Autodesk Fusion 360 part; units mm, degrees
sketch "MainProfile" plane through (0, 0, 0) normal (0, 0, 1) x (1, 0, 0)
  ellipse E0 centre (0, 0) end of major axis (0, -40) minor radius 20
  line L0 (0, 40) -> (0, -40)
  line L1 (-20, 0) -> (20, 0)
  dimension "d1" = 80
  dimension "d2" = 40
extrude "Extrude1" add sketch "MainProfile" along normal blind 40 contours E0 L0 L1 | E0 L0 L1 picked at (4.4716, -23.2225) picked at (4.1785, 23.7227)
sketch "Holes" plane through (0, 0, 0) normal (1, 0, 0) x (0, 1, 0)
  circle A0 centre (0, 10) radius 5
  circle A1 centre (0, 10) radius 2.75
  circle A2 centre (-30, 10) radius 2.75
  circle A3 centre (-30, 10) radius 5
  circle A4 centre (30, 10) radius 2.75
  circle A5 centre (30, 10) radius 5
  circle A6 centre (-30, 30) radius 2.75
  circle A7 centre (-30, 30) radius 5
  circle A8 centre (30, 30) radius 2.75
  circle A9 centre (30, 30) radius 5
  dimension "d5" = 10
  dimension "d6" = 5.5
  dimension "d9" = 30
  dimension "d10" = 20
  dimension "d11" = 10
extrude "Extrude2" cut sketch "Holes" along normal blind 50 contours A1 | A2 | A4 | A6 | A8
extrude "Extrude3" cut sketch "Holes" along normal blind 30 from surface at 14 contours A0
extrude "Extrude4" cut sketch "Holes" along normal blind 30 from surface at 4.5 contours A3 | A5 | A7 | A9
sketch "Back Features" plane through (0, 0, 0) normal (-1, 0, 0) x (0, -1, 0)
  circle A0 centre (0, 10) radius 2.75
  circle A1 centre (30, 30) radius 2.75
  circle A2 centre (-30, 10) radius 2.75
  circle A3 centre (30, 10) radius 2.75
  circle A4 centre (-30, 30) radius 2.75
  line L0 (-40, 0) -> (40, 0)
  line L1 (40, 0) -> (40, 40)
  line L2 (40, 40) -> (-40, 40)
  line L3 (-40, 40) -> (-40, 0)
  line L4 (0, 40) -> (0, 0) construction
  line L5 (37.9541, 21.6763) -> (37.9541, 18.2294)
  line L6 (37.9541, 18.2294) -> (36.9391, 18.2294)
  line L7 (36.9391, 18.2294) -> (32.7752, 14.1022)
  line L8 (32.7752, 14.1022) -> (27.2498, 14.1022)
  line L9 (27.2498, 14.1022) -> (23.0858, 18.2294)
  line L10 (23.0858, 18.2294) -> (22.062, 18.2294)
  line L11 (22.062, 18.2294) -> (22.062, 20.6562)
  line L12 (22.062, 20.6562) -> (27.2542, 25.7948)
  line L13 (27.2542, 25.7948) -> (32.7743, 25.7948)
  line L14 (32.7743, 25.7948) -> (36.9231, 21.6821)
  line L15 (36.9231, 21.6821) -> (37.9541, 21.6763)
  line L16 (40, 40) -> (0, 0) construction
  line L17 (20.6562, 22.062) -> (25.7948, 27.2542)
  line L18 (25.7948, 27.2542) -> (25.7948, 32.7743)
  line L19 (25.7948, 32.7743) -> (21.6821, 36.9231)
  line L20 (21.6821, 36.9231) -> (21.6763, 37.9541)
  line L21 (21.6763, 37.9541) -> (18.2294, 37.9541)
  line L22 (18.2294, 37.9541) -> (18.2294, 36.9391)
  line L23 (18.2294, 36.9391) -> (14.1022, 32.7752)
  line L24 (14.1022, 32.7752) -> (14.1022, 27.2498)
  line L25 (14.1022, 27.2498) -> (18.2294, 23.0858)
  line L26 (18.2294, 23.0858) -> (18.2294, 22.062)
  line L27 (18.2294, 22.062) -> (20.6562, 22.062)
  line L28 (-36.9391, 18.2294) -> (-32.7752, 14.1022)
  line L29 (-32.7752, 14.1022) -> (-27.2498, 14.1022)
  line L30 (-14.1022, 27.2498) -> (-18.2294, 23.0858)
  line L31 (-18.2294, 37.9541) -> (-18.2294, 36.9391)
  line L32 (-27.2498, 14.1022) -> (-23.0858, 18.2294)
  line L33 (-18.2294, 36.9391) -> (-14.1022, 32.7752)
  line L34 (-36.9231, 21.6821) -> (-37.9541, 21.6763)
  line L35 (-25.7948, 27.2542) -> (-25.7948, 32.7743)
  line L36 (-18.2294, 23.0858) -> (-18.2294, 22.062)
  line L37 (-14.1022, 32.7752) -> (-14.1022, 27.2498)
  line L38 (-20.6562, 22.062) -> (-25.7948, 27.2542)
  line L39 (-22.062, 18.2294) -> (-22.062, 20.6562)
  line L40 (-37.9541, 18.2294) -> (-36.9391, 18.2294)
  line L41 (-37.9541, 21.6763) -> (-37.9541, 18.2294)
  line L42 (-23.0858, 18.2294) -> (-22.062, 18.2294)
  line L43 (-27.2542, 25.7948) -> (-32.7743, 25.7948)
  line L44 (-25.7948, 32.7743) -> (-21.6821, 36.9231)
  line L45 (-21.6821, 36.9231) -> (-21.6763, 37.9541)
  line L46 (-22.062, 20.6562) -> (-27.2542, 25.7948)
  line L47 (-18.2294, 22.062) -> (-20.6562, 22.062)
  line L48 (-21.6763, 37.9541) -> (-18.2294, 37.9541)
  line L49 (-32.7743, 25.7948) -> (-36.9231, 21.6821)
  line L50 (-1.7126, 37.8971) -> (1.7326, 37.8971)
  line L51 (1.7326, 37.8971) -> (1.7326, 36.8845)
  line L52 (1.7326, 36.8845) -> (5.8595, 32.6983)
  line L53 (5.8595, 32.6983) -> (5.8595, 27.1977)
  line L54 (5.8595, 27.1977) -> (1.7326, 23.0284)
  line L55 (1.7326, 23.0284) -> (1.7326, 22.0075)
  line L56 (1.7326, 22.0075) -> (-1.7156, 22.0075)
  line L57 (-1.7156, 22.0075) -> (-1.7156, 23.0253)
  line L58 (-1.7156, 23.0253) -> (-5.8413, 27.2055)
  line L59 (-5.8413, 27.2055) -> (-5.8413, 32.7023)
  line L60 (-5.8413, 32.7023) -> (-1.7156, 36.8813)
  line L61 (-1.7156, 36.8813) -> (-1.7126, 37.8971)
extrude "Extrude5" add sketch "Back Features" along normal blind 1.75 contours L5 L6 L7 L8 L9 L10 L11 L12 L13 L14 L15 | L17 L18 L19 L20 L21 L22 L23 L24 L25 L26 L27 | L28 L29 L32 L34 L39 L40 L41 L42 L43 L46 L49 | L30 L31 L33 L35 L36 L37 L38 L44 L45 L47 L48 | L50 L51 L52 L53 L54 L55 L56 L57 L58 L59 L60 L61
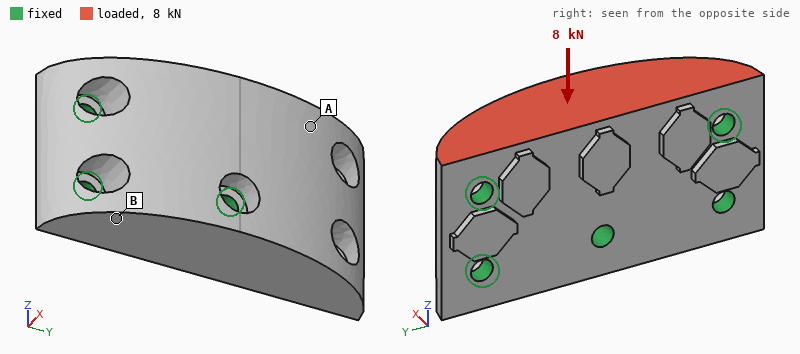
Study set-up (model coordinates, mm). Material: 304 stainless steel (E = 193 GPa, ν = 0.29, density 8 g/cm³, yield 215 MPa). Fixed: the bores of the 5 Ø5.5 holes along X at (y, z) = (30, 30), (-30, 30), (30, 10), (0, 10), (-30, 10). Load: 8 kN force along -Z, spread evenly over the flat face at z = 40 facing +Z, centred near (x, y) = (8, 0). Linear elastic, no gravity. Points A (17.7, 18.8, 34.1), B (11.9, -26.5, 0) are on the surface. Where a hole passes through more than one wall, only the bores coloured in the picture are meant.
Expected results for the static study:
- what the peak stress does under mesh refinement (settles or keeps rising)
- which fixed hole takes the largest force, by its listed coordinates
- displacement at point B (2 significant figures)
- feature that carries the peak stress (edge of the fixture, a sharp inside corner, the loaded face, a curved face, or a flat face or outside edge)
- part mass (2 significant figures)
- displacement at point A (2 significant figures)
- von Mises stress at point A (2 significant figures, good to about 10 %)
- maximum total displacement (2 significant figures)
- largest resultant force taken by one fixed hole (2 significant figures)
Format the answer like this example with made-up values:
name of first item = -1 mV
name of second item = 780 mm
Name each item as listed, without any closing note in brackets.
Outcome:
what the peak stress does under mesh refinement = keeps rising
which fixed hole takes the largest force, by its listed coordinates = (0, 10)
displacement at point B = 1.1 µm
feature that carries the peak stress = edge of the fixture
part mass = 380 g
displacement at point A = 2.2 µm
von Mises stress at point A = 7.6 MPa
maximum total displacement = 2.8 µm
largest resultant force taken by one fixed hole = 3.9 kN
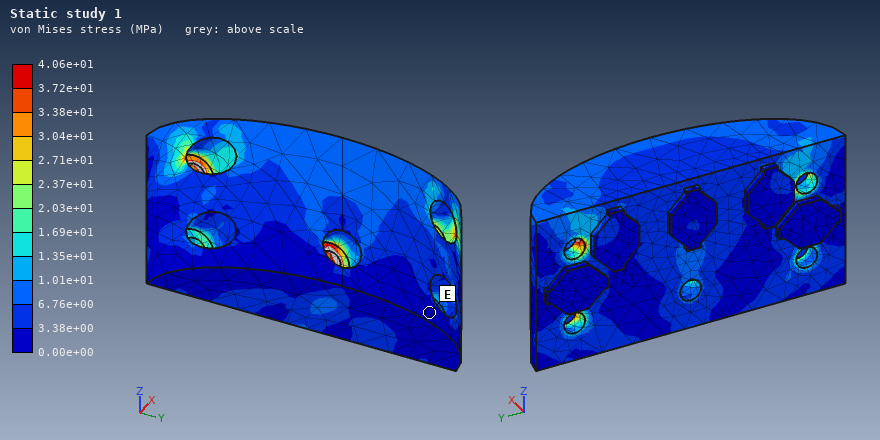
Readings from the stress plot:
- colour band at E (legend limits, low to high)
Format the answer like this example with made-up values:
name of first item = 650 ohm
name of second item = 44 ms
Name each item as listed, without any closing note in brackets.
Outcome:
colour band at E = 0.00e+00 to 3.38e+00 MPa
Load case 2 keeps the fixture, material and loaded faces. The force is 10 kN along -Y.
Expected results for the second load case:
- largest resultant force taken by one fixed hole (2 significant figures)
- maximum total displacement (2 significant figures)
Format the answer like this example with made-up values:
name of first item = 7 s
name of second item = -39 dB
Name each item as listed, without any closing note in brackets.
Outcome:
largest resultant force taken by one fixed hole = 3.6 kN
maximum total displacement = 4.5 µm
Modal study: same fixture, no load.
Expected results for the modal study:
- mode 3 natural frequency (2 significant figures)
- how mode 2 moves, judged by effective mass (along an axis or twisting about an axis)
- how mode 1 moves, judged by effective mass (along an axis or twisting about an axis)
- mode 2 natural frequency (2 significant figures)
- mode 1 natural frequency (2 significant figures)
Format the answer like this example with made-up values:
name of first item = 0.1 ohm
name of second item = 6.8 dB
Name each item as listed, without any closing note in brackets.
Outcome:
mode 3 natural frequency = 26 kHz
how mode 2 moves, judged by effective mass = along Y
how mode 1 moves, judged by effective mass = along X
mode 2 natural frequency = 24 kHz
mode 1 natural frequency = 14 kHz
